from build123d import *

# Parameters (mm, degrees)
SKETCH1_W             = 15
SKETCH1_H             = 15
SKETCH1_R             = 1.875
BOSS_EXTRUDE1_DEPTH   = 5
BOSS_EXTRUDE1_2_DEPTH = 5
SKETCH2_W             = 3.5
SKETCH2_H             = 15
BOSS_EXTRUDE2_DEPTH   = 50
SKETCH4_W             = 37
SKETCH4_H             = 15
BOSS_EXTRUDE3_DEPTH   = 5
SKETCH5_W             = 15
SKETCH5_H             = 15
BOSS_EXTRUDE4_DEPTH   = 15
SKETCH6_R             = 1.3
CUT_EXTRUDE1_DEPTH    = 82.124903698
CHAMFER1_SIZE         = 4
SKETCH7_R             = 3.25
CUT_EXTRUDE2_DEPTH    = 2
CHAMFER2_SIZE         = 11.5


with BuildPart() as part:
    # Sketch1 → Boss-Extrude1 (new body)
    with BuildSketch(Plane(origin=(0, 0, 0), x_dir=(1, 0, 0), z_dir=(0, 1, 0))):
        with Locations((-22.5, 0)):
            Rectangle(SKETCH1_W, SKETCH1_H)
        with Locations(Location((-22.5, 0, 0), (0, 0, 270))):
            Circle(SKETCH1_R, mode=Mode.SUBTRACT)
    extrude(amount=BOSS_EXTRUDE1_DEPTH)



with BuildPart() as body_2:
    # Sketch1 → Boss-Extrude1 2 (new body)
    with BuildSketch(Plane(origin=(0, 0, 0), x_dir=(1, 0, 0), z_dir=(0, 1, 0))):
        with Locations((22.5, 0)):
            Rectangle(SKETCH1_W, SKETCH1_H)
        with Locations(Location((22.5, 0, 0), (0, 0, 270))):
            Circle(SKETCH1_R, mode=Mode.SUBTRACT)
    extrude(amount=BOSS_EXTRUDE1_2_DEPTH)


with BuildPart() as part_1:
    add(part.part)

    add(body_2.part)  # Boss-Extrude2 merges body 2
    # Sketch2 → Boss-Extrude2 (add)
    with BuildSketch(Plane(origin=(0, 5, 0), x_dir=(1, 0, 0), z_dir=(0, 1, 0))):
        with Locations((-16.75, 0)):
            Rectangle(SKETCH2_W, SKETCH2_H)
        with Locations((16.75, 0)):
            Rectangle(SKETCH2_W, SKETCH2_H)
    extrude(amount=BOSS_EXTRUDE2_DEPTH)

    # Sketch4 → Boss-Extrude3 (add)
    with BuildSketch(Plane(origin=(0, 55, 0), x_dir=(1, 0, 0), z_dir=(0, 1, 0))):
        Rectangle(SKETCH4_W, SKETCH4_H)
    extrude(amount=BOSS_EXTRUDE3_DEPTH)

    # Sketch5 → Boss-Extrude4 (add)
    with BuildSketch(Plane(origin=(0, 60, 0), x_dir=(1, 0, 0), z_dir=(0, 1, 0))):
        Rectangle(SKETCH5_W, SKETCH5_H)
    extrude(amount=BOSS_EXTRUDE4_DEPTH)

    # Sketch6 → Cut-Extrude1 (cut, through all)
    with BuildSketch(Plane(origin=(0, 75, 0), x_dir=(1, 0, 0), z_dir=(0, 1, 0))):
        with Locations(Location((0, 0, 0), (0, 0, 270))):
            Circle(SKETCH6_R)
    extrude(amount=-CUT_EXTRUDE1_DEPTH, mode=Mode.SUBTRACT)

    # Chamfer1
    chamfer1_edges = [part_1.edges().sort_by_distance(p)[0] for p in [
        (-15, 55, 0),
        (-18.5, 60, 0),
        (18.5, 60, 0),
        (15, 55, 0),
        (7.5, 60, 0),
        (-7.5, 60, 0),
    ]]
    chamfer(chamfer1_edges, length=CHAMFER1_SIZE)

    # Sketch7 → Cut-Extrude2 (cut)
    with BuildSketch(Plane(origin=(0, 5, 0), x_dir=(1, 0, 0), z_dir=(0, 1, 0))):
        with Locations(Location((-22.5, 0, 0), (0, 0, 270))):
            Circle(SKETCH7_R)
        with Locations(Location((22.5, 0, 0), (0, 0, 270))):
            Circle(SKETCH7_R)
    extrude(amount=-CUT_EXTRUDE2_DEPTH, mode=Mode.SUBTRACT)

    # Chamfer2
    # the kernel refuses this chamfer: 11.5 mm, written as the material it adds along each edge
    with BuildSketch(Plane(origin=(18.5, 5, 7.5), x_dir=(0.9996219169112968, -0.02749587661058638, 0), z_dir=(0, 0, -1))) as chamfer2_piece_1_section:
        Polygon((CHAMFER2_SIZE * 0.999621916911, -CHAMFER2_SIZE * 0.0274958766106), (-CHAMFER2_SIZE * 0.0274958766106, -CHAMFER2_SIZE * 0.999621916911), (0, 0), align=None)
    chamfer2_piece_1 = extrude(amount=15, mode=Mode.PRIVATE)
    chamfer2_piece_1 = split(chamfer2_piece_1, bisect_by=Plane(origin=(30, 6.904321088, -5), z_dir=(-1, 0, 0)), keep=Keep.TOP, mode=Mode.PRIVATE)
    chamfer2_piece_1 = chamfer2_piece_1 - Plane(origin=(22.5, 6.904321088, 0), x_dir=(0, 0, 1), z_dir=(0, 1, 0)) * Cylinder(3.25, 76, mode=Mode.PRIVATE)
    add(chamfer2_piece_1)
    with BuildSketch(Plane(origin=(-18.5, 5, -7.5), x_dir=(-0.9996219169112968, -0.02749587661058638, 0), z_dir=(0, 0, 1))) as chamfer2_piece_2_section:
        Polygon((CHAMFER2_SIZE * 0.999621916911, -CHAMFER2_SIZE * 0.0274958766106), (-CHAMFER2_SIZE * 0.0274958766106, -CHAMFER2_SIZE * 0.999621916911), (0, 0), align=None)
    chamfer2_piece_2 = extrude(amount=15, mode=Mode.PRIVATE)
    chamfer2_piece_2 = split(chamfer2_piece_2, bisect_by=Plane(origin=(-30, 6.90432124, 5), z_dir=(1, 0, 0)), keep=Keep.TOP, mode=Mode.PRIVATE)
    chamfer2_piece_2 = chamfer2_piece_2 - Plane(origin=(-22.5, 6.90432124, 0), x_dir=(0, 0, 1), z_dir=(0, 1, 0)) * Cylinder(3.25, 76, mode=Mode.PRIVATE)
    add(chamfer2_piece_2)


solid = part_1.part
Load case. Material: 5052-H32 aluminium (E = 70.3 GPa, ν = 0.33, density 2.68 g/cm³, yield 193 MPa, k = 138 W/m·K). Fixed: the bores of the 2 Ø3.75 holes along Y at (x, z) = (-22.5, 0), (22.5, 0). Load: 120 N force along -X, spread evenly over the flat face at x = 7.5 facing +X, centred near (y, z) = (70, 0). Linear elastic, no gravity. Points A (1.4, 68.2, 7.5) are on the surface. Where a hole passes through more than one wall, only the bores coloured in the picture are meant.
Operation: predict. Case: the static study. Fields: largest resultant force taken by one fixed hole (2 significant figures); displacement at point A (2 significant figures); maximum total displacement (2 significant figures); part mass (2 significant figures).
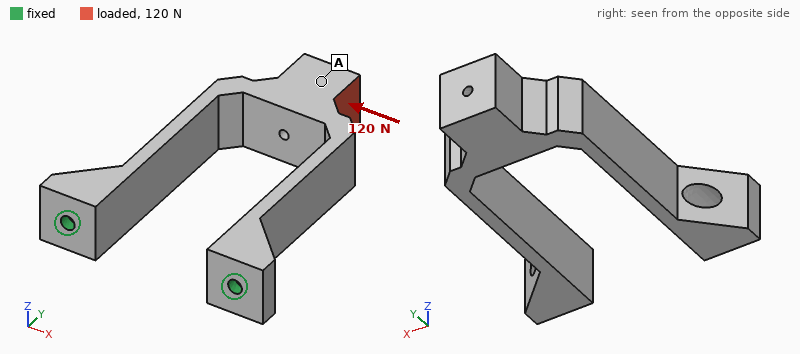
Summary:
140 N
0.098 mm
0.10 mm
40 g
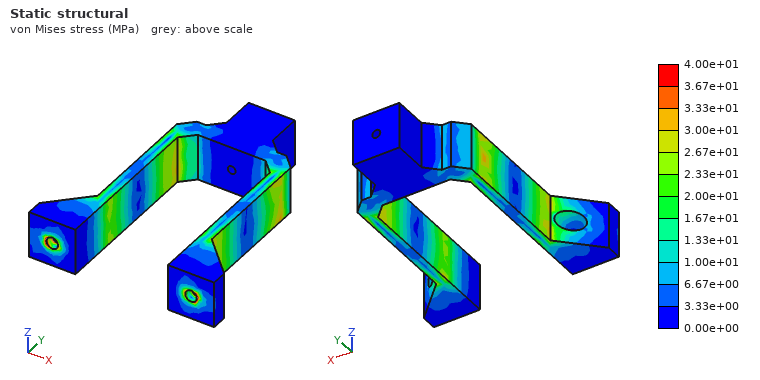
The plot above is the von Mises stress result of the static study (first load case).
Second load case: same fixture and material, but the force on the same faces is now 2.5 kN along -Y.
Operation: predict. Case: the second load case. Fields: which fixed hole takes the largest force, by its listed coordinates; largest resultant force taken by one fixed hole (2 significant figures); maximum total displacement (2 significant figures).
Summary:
(22.5, 0)
1.8 kN
81 µm
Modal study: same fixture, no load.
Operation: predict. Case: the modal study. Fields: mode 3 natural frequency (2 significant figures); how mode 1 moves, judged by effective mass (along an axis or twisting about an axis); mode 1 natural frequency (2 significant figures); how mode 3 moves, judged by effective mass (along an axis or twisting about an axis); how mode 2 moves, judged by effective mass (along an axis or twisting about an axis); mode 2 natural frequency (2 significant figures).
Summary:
3100 Hz
along Z
1000 Hz
twisting about Y
along X
1200 Hz
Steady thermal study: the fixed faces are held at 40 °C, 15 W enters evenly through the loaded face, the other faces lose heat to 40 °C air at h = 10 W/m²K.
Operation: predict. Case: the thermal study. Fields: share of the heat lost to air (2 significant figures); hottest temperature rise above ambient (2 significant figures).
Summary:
13 %
58 K
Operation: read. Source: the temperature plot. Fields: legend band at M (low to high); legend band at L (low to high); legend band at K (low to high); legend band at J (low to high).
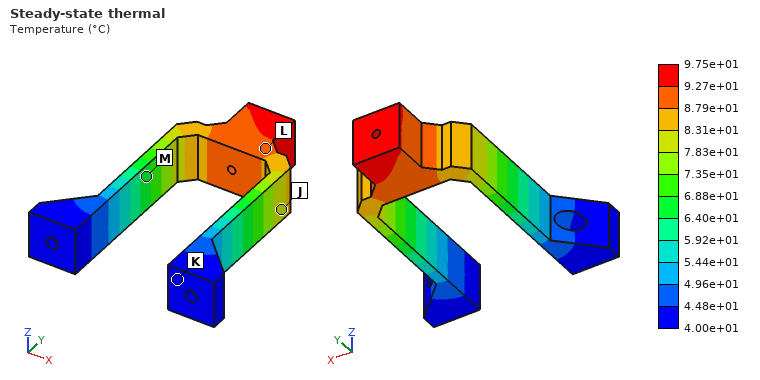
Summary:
6.40e+01 to 6.88e+01 °C
8.79e+01 to 9.27e+01 °C
4.00e+01 to 4.48e+01 °C
7.83e+01 to 8.31e+01 °C
